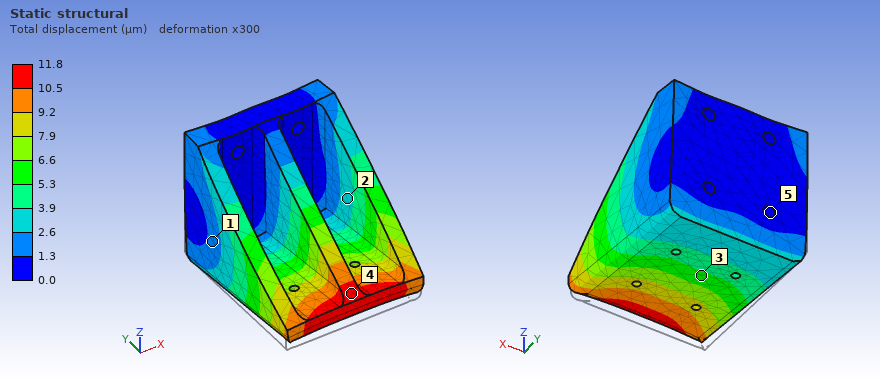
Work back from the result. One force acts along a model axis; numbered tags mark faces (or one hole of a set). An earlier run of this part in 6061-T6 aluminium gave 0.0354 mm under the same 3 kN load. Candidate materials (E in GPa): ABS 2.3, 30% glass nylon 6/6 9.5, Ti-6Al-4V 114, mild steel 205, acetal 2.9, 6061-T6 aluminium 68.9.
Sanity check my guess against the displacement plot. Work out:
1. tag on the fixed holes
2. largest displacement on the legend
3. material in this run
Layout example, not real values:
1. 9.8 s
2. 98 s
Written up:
1. 5
2. 11.8 µm
3. mild steel
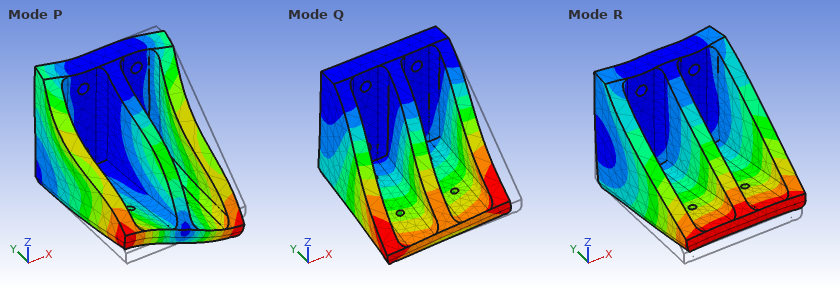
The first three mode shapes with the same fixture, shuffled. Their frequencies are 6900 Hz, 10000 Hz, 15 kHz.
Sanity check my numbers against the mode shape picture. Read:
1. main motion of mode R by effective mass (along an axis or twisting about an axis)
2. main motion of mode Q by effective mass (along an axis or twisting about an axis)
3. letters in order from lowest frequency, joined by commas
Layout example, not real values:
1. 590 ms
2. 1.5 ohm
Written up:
1. along Z
2. along X
3. Q, R, P
